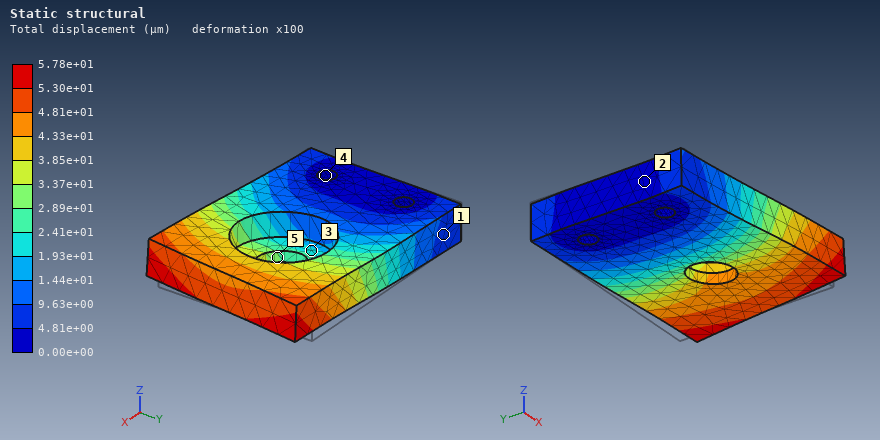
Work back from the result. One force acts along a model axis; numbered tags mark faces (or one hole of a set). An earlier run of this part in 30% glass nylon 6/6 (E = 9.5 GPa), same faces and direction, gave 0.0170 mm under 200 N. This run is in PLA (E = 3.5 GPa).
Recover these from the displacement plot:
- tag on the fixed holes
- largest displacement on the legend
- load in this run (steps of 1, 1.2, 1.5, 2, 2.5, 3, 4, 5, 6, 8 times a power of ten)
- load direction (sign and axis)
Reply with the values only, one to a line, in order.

4
5.78e+01 µm
250 N
-Y
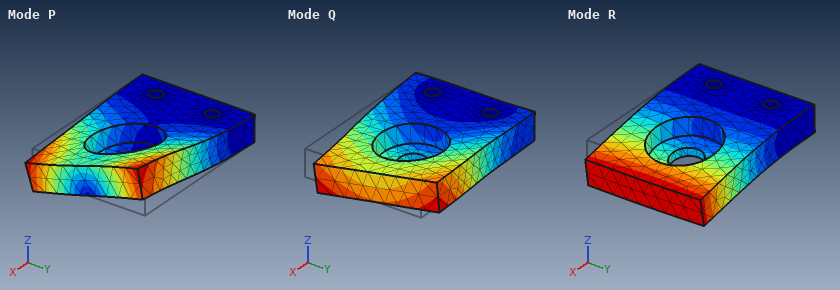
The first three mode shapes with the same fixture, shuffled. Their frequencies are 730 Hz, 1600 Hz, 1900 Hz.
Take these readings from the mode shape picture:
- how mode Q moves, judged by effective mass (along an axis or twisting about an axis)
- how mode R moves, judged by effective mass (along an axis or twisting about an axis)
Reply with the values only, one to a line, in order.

along Y
along Z
